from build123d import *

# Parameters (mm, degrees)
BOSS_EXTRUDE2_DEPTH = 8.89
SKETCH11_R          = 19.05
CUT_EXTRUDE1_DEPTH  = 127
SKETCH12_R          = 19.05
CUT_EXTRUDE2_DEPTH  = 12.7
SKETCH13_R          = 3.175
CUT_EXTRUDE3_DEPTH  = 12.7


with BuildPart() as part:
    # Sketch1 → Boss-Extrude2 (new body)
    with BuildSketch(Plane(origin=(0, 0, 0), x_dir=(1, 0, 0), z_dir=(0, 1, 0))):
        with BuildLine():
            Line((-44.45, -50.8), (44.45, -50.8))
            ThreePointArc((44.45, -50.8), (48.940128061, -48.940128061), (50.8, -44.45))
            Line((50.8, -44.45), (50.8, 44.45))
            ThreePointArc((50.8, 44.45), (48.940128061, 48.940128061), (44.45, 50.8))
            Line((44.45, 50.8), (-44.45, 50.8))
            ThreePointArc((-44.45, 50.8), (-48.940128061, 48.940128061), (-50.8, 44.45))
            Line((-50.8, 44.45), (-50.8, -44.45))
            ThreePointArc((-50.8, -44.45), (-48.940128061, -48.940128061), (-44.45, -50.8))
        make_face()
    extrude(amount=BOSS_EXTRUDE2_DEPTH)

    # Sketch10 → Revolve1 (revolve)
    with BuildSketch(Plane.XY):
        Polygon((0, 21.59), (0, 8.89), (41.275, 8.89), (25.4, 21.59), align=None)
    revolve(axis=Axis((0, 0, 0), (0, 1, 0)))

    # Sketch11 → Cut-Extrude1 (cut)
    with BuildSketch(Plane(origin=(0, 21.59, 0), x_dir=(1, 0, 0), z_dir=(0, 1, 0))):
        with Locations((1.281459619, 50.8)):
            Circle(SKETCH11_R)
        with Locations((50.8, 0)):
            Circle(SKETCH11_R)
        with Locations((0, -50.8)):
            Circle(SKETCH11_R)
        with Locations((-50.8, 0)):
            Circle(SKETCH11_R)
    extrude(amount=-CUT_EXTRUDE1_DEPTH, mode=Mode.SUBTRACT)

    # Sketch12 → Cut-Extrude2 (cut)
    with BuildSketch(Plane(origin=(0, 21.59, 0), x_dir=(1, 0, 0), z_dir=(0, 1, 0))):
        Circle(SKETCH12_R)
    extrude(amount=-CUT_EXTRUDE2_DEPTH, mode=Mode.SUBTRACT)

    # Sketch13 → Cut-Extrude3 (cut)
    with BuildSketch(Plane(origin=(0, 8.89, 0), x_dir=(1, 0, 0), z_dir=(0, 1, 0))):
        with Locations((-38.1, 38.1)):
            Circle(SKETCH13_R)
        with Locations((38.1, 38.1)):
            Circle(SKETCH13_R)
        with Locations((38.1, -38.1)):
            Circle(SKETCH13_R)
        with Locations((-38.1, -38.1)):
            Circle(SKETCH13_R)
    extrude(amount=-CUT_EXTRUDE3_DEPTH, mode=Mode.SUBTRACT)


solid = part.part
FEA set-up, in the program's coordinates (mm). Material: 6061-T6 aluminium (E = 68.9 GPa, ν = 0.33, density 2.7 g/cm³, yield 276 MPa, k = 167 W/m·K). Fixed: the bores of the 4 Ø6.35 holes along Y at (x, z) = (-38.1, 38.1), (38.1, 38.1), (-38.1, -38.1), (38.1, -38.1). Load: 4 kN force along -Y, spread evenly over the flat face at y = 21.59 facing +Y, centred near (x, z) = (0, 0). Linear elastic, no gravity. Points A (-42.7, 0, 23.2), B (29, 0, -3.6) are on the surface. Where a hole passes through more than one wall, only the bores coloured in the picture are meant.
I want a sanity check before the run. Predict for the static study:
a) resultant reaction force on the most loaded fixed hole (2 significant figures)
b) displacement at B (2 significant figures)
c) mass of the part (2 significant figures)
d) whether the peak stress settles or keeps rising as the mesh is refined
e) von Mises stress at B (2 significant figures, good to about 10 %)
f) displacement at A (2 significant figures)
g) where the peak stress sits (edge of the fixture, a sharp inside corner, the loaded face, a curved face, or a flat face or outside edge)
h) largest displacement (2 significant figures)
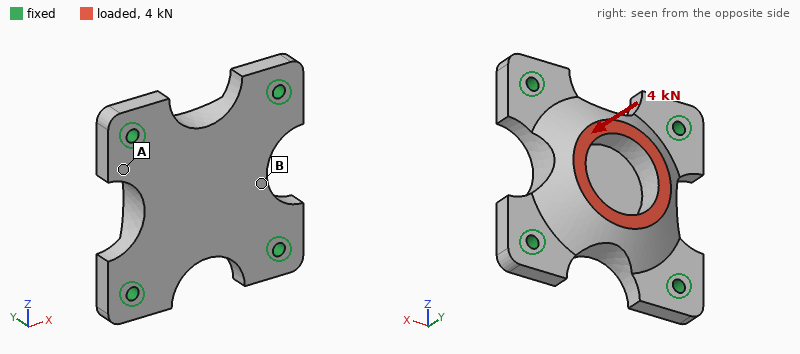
1.2 kN
14 µm
270 g
keeps rising
8.4 MPa
5.5 µm
edge of the fixture
18 µm
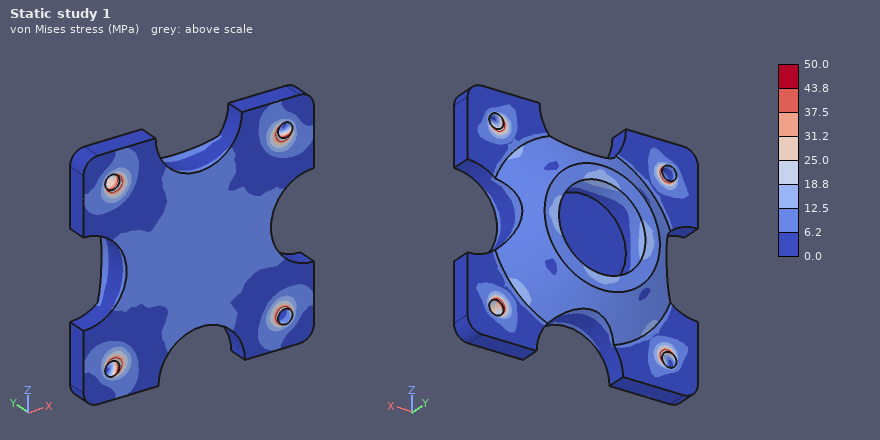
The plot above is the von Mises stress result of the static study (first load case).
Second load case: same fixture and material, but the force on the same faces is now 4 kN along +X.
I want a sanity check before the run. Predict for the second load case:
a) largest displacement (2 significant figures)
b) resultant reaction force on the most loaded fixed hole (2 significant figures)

8.6 µm
1.3 kN
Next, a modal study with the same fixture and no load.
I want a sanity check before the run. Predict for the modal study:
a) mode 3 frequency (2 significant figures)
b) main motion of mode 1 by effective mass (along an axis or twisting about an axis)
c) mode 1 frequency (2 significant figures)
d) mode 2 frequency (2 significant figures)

10 kHz
along Y
6200 Hz
10 kHz
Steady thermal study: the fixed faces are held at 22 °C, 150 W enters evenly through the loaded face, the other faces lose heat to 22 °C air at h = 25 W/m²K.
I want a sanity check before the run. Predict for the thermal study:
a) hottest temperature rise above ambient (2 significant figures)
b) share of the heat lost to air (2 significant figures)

27 K
4.6 %
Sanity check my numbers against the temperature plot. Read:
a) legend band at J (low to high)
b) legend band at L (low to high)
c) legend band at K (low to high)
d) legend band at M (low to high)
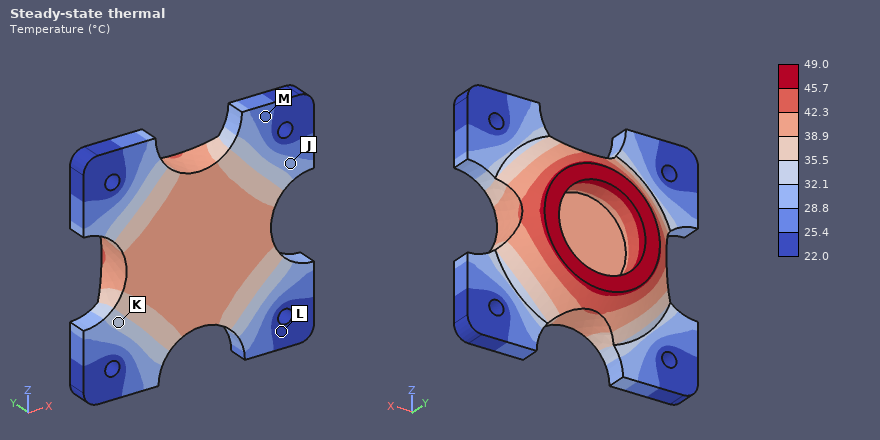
28.8 to 32.1 °C
22.0 to 25.4 °C
32.1 to 35.5 °C
25.4 to 28.8 °C
